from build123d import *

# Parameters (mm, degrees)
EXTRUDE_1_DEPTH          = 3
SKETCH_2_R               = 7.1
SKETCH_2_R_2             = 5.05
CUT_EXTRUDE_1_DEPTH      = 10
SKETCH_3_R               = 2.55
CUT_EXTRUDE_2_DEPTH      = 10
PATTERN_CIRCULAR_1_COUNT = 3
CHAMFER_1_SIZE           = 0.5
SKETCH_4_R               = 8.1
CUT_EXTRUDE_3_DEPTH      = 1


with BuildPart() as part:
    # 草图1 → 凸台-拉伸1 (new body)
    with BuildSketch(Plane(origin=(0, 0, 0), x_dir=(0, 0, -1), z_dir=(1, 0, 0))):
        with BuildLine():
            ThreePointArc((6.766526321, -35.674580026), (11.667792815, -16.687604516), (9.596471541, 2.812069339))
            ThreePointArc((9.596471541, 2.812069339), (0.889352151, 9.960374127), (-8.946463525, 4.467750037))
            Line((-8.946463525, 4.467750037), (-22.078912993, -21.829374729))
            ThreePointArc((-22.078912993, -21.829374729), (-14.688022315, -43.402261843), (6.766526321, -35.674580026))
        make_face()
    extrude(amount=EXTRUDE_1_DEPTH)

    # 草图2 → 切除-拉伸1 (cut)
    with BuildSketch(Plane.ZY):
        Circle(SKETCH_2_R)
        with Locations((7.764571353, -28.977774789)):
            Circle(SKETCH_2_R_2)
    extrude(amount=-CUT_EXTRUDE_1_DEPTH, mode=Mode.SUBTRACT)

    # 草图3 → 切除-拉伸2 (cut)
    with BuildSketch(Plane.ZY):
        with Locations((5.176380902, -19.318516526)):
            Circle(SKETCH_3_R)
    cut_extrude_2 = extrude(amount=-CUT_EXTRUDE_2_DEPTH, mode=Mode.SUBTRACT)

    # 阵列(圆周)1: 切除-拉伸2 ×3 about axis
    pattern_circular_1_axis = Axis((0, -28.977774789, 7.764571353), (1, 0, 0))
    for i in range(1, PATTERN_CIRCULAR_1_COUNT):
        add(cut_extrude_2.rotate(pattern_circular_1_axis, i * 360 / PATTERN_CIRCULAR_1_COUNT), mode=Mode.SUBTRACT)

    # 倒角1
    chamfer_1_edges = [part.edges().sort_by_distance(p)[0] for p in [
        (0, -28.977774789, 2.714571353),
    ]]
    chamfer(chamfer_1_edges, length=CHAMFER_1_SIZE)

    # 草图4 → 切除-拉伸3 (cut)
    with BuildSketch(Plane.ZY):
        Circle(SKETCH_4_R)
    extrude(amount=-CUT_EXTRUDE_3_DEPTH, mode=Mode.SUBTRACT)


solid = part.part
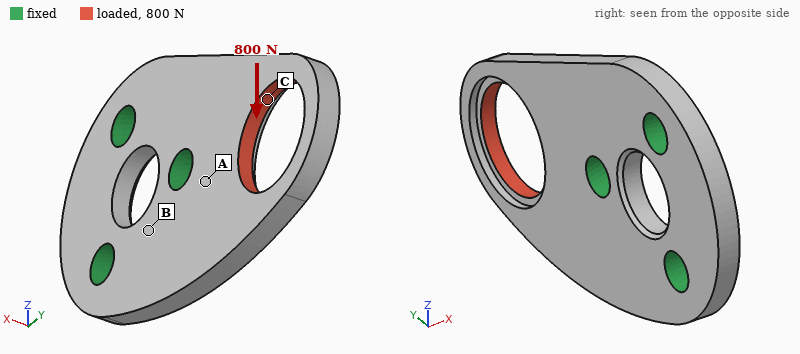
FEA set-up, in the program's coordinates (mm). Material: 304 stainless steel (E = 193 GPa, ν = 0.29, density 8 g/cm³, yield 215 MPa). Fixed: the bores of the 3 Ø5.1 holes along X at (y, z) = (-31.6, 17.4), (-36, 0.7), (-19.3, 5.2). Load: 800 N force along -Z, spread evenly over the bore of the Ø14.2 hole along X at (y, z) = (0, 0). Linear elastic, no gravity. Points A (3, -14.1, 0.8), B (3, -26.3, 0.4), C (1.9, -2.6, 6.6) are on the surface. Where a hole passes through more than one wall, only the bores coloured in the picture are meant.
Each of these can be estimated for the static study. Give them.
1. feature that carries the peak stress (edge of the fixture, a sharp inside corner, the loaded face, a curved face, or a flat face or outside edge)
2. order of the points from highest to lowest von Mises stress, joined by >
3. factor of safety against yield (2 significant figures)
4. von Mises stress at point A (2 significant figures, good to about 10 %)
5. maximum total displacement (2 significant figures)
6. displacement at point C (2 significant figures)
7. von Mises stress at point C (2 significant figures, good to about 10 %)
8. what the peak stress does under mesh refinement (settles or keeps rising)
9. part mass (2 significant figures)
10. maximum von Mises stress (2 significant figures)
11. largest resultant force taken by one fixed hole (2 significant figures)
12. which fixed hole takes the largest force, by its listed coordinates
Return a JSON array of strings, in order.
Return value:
["the loaded face", "C > A > B", "1.4", "40 MPa", "25 µm", "7.2 µm", "120 MPa", "settles", "26 g", "160 MPa", "1.0 kN", "(-19.3, 5.2)"]
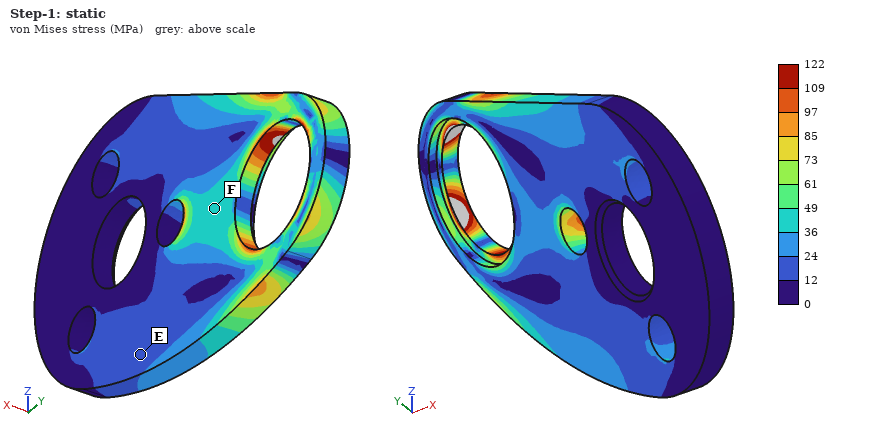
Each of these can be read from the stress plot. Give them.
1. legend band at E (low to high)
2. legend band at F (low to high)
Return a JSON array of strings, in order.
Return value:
["12 to 24 MPa", "36 to 49 MPa"]
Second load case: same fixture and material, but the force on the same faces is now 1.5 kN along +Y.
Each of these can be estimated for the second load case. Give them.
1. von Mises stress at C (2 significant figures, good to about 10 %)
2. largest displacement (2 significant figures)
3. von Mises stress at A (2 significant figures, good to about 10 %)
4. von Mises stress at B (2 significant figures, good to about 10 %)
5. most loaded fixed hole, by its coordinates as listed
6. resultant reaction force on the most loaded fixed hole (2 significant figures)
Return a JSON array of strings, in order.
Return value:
["59 MPa", "34 µm", "31 MPa", "14 MPa", "(-19.3, 5.2)", "960 N"]
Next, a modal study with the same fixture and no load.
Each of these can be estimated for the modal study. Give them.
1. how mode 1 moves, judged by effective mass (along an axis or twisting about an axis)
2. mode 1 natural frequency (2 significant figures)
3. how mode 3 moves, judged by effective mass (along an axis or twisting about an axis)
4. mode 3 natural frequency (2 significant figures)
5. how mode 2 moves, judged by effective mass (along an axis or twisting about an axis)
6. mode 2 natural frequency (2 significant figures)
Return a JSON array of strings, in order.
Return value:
["along X", "4400 Hz", "along X", "13 kHz", "twisting about Y", "7700 Hz"]
